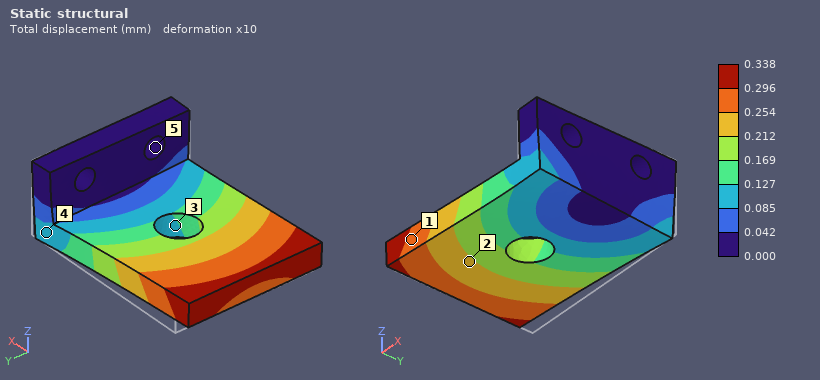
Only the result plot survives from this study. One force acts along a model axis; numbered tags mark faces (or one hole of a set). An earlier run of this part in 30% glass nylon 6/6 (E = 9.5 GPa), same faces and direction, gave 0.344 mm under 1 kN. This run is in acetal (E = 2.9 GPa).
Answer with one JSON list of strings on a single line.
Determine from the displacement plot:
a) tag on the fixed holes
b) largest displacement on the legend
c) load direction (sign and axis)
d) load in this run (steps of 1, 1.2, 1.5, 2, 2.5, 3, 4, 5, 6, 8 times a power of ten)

["5", "0.338 mm", "-Y", "300 N"]
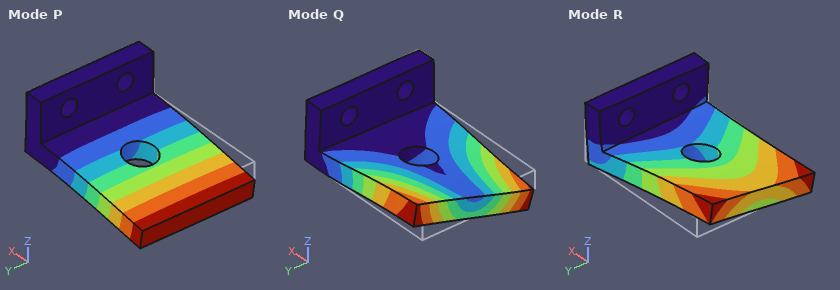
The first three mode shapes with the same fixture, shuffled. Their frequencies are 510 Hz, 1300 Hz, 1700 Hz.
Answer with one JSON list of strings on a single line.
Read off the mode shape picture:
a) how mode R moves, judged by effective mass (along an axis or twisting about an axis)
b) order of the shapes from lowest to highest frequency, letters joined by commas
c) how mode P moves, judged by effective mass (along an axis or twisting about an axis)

["along Y", "P, R, Q", "along Z"]
